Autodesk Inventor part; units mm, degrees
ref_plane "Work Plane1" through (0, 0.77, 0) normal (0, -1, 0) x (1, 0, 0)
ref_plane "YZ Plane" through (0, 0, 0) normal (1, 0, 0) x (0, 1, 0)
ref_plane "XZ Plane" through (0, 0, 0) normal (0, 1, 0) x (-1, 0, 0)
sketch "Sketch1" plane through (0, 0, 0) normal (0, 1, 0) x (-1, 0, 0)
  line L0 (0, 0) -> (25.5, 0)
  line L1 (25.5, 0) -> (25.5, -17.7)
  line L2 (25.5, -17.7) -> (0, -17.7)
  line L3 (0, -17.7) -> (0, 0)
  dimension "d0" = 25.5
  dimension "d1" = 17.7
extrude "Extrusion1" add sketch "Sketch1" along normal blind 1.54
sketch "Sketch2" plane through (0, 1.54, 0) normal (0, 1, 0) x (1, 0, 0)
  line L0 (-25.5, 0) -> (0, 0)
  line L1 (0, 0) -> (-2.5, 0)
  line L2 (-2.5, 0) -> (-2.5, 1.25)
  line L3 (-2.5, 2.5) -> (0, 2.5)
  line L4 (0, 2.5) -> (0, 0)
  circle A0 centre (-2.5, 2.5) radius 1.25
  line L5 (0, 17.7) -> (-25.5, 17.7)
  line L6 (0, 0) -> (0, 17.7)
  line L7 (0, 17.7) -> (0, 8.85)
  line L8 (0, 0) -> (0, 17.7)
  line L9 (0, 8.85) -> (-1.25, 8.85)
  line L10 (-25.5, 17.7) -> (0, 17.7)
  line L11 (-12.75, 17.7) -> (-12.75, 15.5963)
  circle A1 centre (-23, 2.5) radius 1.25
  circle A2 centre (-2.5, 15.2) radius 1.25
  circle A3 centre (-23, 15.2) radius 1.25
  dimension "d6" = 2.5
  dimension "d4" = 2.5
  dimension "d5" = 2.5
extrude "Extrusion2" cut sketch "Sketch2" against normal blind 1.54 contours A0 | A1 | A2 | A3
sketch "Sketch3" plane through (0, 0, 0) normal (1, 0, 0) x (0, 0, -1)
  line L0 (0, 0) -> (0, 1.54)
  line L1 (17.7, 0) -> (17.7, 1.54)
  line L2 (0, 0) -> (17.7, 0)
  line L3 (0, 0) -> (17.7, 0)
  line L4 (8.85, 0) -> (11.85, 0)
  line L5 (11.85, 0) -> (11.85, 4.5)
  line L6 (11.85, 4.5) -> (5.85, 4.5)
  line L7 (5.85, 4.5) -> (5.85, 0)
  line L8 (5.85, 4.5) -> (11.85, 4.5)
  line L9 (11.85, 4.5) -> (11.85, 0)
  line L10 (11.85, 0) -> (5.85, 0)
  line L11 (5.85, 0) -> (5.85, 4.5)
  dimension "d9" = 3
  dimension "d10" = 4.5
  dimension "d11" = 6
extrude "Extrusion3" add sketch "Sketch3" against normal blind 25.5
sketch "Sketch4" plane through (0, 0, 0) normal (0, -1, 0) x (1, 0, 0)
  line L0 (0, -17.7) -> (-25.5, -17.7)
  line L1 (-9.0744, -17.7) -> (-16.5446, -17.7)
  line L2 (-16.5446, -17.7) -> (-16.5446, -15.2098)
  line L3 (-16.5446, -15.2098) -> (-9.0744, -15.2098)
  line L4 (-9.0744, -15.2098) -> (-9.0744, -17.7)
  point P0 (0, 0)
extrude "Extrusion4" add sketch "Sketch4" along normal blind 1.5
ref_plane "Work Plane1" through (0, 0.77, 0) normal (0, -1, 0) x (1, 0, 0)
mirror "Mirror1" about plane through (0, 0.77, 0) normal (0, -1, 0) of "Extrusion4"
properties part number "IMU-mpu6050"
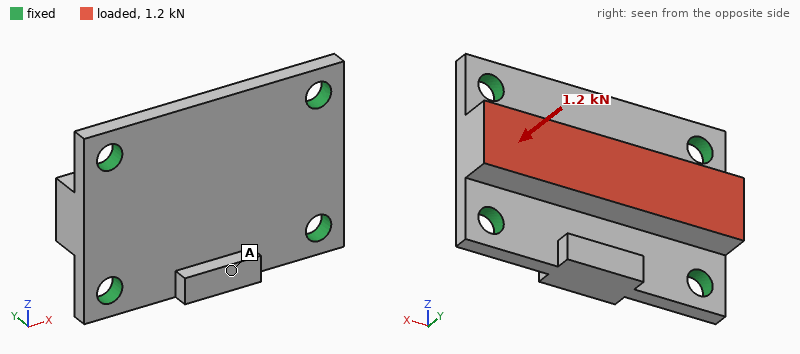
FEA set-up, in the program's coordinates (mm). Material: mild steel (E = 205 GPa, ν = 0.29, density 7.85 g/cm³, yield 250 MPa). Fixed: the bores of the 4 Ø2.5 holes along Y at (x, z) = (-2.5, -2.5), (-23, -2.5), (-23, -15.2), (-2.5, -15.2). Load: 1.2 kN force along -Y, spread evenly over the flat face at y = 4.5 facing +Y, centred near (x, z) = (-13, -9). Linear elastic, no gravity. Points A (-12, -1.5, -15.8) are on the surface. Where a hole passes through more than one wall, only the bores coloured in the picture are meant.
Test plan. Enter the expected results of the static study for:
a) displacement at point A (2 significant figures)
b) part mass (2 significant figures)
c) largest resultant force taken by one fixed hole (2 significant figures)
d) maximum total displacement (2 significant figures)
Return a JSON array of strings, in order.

["4.7 µm", "9.2 g", "340 N", "7.9 µm"]
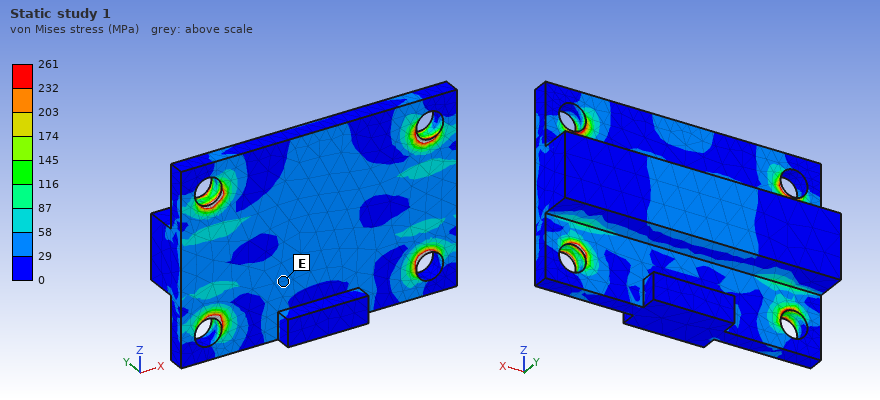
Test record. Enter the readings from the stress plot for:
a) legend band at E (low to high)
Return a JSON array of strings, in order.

["29 to 58 MPa"]
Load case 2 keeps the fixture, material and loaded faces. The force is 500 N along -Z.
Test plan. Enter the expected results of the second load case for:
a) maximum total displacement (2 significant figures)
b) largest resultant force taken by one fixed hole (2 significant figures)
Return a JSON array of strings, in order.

["2.3 µm", "170 N"]
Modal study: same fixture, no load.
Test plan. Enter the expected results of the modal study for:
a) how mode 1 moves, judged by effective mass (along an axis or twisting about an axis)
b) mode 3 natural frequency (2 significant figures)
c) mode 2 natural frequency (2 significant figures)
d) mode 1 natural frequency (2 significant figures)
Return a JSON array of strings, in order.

["along Y", "40 kHz", "29 kHz", "24 kHz"]
